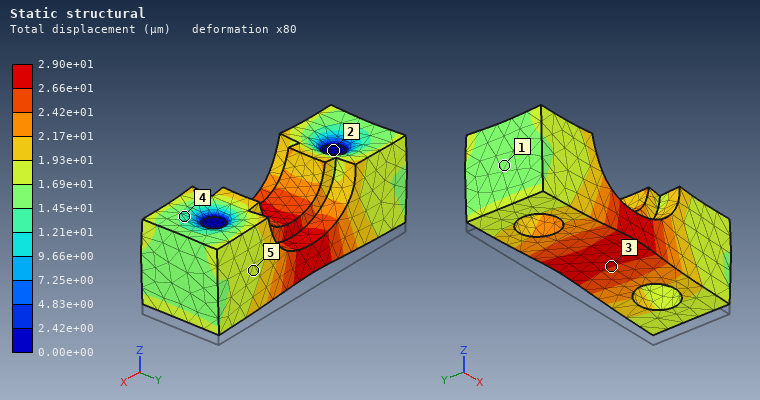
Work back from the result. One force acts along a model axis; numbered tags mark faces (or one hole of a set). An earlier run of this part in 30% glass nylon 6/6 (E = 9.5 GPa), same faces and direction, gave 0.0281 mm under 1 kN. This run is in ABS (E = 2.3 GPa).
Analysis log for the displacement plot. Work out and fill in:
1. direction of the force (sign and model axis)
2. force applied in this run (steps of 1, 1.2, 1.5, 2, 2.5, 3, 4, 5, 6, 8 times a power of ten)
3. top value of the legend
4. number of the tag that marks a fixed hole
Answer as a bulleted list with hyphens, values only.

- +Z
- 250 N
- 2.90e+01 µm
- 2
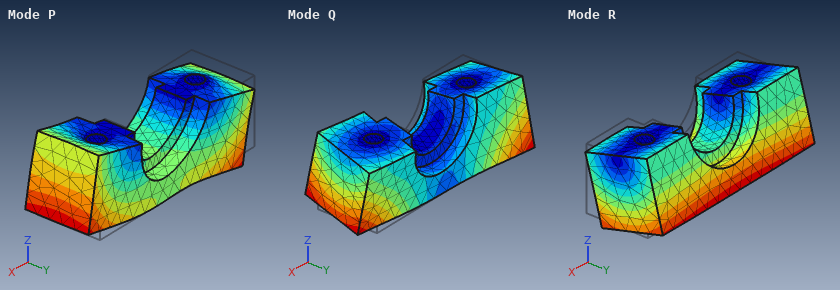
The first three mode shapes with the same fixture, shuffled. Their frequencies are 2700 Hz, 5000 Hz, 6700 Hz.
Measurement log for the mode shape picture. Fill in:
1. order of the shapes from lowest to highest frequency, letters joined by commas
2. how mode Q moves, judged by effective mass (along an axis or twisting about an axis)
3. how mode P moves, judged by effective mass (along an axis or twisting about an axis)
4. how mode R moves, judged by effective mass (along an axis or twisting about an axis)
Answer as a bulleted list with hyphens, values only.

- R, Q, P
- twisting about Z
- along X
- along Y
